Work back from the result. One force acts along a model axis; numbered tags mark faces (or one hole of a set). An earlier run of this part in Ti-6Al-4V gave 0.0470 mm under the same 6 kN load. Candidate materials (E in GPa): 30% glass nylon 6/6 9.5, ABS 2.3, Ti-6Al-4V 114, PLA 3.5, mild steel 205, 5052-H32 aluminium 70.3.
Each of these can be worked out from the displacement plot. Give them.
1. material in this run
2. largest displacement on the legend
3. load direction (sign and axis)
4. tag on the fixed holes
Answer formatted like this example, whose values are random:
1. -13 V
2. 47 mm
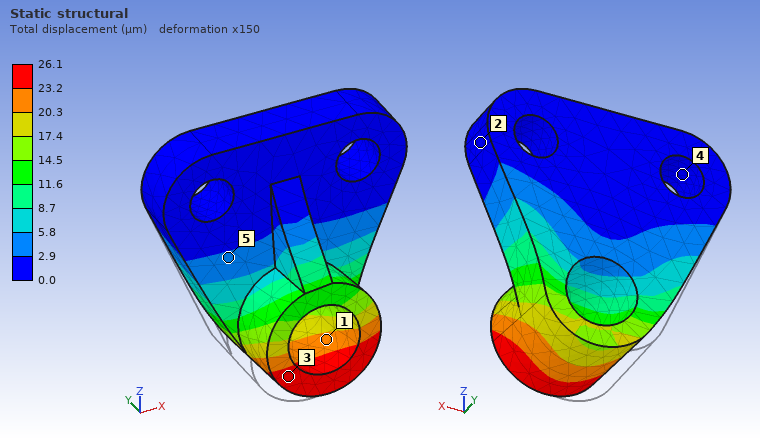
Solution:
1. mild steel
2. 26.1 µm
3. +X
4. 4
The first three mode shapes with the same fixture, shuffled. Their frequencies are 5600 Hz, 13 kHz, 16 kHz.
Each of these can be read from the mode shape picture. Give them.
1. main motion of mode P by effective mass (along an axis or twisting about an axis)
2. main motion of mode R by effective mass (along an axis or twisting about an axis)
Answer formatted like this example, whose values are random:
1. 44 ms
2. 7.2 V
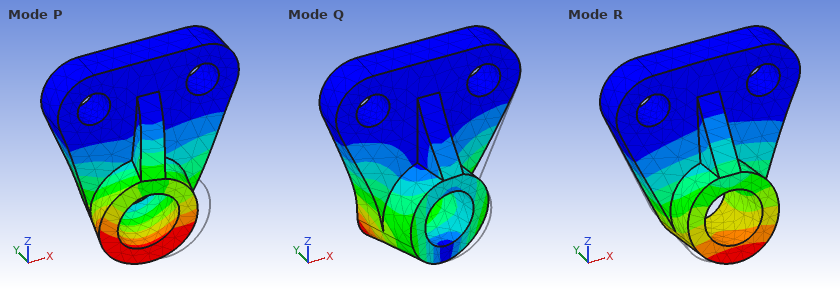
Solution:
1. along X
2. along Y
